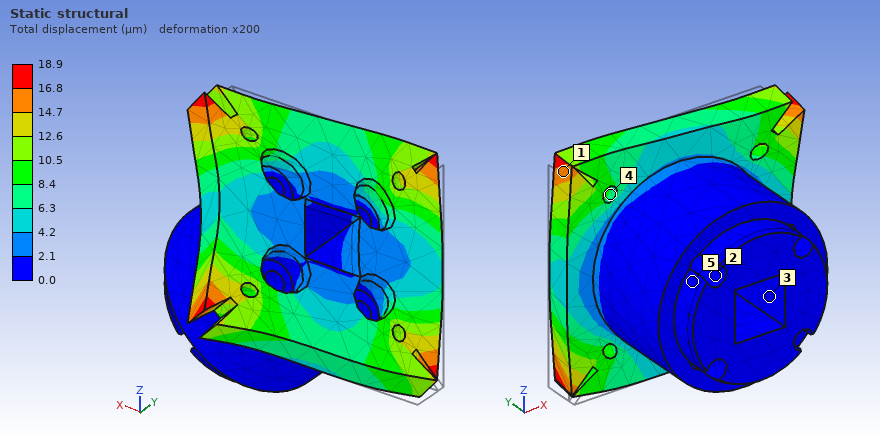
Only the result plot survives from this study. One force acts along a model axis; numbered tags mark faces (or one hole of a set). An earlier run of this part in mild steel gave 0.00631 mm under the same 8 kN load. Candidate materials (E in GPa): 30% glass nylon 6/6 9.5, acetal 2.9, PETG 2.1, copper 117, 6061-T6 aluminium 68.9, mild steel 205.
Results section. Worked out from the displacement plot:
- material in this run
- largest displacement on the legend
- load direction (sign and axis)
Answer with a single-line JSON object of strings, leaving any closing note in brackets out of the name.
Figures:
{"material in this run": "6061-T6 aluminium", "largest displacement on the legend": "18.9 µm", "load direction": "+X"}
